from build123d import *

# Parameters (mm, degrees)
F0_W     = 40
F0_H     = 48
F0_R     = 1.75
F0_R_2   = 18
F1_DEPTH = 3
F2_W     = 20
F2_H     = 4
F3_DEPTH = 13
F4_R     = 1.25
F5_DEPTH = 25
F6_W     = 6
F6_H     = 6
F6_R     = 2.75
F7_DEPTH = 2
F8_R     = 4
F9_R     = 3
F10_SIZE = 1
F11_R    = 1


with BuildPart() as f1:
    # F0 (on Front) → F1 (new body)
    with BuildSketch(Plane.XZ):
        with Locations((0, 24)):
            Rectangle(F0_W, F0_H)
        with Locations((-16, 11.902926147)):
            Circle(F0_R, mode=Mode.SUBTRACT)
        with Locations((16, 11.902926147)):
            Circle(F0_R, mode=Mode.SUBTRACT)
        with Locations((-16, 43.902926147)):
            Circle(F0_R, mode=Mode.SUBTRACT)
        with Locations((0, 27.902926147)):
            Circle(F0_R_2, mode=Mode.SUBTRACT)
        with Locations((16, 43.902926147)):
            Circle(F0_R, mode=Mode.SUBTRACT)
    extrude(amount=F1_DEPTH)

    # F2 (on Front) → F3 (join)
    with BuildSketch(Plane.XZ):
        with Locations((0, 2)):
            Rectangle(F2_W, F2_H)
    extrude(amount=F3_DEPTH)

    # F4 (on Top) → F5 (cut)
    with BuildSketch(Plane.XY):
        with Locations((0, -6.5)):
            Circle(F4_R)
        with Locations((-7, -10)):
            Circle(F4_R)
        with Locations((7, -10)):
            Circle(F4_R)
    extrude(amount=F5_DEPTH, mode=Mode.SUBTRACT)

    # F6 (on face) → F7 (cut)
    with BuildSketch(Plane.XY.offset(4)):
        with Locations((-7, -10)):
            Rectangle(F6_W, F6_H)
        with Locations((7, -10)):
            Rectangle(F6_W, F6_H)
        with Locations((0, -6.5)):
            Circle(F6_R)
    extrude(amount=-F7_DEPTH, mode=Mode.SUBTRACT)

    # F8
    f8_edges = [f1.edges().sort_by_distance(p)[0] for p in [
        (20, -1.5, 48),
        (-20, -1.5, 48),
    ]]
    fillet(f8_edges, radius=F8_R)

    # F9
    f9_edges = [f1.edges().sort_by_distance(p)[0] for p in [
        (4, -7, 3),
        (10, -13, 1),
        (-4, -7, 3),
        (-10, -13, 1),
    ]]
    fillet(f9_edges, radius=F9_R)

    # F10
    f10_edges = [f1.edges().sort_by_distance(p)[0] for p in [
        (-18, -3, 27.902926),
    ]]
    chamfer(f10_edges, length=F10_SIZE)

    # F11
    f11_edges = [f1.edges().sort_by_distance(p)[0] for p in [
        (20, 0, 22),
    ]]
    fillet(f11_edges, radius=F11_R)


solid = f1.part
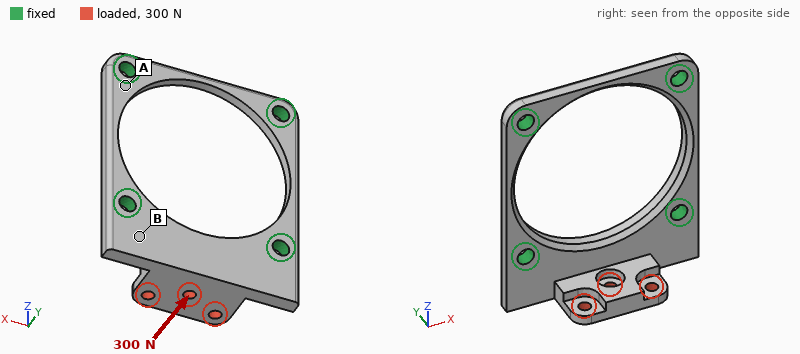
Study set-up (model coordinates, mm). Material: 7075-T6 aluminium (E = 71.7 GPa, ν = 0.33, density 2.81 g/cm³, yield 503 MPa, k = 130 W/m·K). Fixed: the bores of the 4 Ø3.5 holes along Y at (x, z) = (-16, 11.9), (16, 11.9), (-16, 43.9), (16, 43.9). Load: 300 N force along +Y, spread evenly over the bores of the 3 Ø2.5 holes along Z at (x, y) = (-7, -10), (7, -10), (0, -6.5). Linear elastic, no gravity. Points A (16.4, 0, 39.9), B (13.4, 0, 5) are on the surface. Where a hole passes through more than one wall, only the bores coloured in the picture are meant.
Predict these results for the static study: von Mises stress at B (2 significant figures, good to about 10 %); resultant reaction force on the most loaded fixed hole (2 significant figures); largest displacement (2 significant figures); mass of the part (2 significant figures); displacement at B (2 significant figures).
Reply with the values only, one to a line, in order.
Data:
35 MPa
150 N
76 µm
8.6 g
19 µm
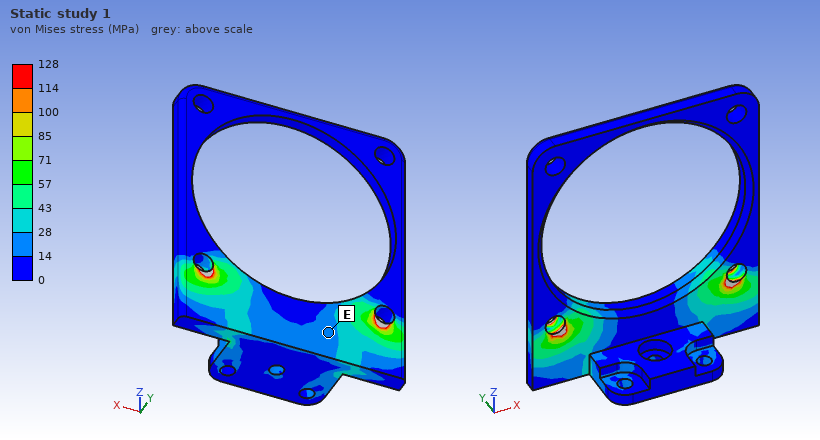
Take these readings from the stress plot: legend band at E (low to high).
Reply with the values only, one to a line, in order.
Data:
14 to 28 MPa
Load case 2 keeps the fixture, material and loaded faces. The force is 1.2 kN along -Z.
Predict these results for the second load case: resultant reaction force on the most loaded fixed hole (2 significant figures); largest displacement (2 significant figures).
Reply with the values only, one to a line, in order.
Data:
810 N
0.37 mm
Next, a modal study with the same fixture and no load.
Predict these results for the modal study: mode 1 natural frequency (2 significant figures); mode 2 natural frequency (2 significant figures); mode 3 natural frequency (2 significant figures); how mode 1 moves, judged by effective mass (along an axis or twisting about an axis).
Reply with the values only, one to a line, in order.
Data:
7000 Hz
16 kHz
16 kHz
along Y
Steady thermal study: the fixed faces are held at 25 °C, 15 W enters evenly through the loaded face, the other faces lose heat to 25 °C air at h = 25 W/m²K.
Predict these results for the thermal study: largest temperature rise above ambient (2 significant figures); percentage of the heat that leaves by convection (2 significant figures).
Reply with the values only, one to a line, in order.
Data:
39 K
4.7 %
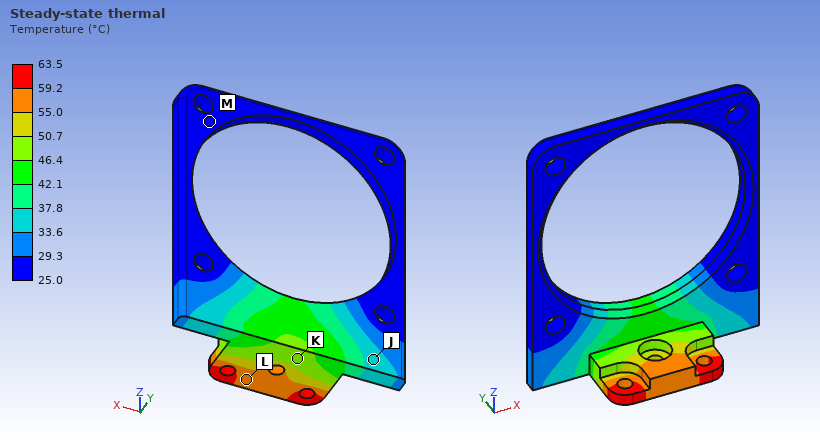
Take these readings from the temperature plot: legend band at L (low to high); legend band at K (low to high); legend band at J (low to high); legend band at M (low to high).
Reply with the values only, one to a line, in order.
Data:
55.0 to 59.2 °C
46.4 to 50.7 °C
33.6 to 37.8 °C
25.0 to 29.3 °C
